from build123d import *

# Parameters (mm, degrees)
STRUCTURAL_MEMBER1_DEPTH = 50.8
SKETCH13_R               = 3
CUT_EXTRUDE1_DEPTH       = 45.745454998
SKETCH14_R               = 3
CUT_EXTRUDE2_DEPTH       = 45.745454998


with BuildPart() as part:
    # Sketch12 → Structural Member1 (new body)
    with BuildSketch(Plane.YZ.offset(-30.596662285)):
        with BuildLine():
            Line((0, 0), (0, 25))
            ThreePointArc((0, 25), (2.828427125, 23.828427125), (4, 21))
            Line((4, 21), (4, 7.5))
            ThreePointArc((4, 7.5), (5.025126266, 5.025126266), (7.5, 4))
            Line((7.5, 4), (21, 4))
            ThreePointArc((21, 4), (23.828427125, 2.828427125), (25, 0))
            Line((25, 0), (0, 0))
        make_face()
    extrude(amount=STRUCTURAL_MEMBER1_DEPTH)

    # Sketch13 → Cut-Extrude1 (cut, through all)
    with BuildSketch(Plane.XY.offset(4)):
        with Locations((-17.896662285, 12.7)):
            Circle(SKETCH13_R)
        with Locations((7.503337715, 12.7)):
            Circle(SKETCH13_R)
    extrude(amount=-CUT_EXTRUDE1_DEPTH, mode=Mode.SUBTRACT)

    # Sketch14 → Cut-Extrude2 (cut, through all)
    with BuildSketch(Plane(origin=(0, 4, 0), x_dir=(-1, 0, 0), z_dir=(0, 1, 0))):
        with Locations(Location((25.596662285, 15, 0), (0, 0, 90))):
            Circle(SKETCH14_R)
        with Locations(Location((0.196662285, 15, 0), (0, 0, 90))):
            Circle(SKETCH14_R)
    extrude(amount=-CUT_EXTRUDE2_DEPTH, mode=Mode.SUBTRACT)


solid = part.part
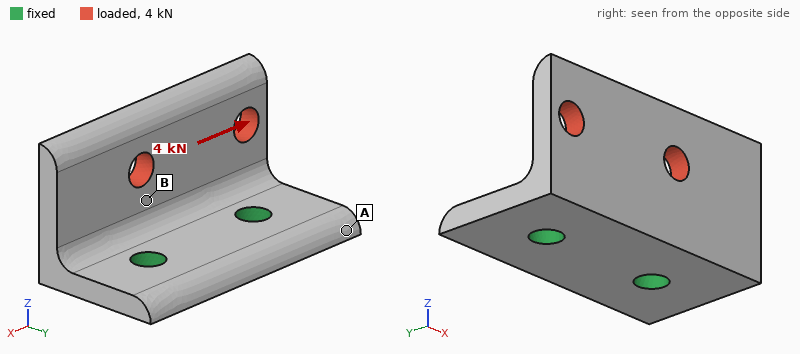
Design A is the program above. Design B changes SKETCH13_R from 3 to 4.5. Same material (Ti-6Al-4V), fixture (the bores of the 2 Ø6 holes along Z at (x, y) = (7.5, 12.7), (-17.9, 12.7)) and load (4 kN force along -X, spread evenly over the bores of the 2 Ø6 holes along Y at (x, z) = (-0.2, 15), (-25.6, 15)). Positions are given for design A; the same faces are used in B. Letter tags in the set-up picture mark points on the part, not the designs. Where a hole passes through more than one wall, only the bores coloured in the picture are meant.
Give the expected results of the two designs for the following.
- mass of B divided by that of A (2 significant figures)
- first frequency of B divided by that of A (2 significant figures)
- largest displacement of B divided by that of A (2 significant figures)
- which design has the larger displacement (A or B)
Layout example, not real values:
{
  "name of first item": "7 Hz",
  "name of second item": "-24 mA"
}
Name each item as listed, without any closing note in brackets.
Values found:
{
  "mass of B divided by that of A": "0.97",
  "first frequency of B divided by that of A": "1.1",
  "largest displacement of B divided by that of A": "0.72",
  "which design has the larger displacement": "A"
}
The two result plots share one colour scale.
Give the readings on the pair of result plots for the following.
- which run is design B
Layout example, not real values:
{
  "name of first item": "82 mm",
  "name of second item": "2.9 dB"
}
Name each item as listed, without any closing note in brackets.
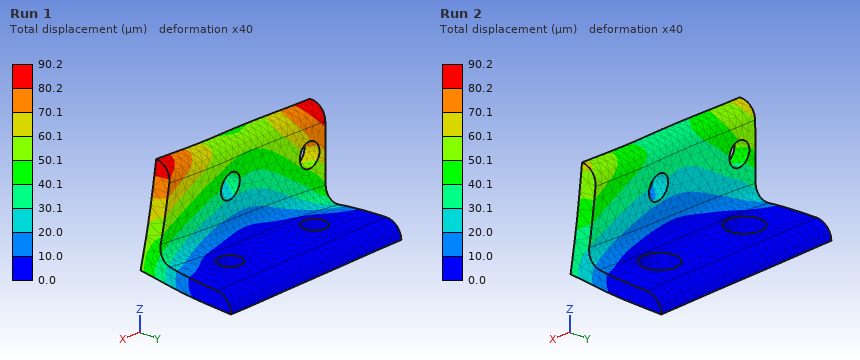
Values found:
{
  "which run is design B": "Run 2"
}
